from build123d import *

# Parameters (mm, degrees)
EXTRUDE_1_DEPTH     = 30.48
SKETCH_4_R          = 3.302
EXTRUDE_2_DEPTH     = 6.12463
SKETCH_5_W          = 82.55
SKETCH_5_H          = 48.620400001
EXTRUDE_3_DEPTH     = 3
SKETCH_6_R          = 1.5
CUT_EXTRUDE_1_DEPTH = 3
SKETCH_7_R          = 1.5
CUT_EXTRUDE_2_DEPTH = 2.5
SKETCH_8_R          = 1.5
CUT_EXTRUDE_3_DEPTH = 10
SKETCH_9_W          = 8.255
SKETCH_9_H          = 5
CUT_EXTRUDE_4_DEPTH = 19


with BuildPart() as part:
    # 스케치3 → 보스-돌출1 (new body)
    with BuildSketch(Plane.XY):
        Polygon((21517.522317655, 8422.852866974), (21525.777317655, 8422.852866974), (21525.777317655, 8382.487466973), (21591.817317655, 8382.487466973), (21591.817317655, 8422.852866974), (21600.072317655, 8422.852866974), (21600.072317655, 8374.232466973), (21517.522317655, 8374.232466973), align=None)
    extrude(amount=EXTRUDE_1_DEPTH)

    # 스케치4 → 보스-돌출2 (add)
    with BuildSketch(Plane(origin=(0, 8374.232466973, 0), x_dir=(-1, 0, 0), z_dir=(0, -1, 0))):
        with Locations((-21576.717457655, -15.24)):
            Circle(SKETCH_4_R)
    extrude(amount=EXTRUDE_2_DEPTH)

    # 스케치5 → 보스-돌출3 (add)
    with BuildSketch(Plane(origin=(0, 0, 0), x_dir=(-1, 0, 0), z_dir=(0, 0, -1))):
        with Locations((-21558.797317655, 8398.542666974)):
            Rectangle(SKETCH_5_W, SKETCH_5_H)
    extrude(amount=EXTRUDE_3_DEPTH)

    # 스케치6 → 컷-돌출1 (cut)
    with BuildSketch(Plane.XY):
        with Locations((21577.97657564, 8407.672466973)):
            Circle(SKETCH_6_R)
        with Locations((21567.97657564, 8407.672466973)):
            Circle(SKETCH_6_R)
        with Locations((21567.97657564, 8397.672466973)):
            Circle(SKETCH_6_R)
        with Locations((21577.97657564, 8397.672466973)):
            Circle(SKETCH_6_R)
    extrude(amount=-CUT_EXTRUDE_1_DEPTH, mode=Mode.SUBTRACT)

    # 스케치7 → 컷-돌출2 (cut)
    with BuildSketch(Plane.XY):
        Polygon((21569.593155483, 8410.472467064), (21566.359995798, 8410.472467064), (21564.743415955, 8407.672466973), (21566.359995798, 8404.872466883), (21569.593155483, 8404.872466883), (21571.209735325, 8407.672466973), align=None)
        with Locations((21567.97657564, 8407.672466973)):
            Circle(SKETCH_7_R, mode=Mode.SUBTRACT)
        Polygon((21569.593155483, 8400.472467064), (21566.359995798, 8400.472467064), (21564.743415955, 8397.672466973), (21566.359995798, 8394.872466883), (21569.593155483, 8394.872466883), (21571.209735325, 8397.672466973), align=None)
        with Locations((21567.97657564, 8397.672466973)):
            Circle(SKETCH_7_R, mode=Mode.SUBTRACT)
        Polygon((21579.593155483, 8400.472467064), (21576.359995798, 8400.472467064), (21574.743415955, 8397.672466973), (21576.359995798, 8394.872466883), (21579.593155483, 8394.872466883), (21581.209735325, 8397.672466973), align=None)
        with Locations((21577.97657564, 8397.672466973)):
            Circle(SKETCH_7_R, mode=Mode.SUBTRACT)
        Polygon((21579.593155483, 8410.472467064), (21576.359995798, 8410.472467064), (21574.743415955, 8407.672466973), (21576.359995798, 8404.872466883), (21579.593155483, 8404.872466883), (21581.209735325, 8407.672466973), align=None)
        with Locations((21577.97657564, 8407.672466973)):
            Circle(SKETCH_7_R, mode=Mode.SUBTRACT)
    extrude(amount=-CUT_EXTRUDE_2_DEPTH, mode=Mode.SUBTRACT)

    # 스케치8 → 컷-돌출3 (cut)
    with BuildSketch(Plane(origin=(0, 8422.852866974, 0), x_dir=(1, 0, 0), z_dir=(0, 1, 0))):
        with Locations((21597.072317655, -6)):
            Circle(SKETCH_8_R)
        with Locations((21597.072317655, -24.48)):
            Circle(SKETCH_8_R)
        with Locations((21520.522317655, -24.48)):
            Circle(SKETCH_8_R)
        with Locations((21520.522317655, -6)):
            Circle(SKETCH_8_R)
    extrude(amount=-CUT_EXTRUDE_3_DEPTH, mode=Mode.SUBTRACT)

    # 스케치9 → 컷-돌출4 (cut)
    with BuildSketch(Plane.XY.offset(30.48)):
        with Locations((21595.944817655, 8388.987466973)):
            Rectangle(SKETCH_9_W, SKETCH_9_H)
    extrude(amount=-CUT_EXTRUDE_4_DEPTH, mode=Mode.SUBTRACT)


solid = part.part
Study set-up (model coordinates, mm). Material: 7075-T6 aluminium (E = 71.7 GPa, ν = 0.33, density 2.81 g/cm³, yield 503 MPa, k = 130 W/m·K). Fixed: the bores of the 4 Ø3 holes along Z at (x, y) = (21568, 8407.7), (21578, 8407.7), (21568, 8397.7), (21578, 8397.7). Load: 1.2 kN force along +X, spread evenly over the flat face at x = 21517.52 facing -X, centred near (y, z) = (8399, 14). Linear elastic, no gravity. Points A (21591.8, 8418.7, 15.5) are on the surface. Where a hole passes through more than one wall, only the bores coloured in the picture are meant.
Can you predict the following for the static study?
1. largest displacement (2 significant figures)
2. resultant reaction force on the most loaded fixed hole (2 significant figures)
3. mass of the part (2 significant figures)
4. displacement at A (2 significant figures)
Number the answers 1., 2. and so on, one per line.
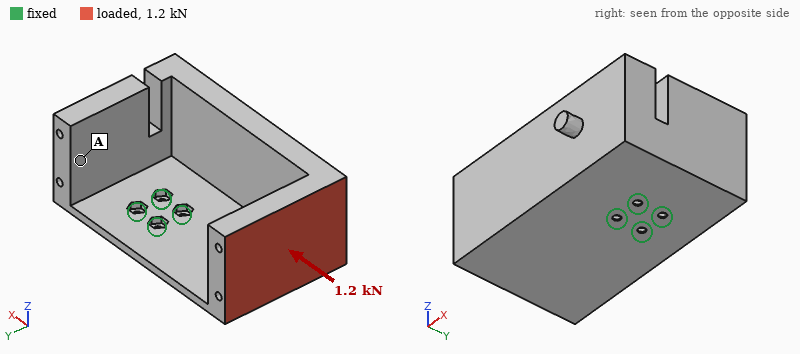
1. 1.0 mm
2. 1.2 kN
3. 150 g
4. 0.33 mm
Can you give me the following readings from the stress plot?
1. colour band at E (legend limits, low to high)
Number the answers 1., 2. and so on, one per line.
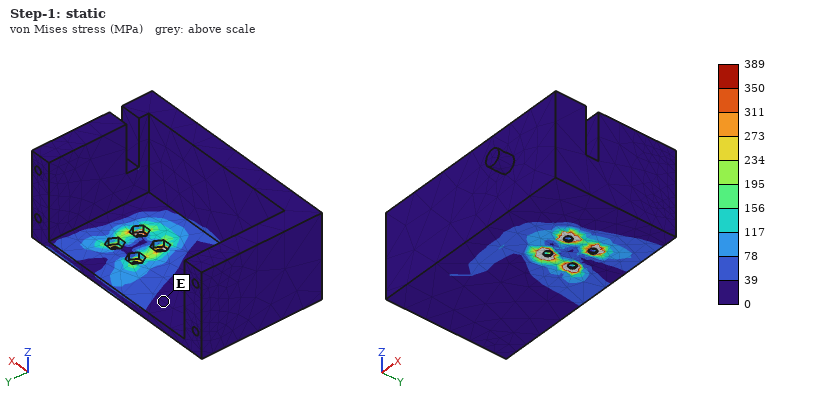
1. 0 to 39 MPa
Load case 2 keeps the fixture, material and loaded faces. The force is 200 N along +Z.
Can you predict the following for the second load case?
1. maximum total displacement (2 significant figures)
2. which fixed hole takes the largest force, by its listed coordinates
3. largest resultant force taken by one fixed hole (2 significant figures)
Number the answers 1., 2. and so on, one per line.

1. 0.60 mm
2. (21568, 8397.7)
3. 710 N
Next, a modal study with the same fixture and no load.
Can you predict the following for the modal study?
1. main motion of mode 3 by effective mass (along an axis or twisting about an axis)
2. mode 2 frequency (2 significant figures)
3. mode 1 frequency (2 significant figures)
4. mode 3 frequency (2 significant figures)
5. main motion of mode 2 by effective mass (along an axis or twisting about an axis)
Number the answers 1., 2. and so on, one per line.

1. along Z
2. 600 Hz
3. 400 Hz
4. 1500 Hz
5. along Y
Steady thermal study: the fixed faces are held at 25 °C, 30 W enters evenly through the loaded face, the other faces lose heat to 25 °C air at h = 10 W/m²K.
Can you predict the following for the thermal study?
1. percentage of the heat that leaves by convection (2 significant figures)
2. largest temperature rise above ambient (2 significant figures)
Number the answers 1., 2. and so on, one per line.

1. 19 %
2. 57 K
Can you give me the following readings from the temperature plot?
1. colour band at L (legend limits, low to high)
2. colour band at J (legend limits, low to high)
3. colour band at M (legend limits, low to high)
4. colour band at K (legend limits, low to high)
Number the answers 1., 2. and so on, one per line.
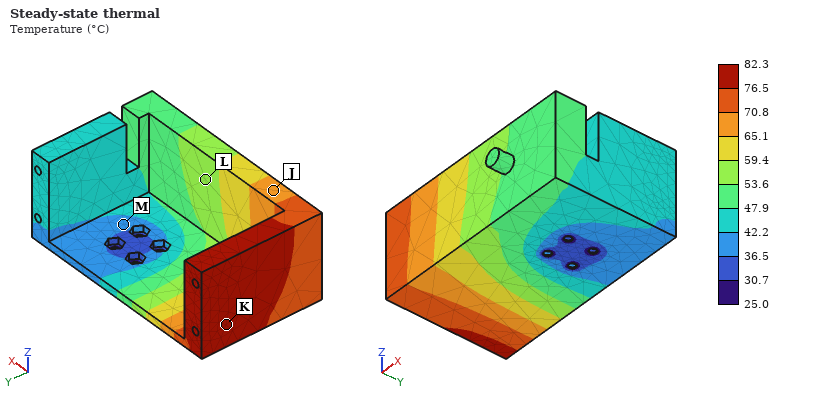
1. 53.6 to 59.4 °C
2. 65.1 to 70.8 °C
3. 36.5 to 42.2 °C
4. 76.5 to 82.3 °C
